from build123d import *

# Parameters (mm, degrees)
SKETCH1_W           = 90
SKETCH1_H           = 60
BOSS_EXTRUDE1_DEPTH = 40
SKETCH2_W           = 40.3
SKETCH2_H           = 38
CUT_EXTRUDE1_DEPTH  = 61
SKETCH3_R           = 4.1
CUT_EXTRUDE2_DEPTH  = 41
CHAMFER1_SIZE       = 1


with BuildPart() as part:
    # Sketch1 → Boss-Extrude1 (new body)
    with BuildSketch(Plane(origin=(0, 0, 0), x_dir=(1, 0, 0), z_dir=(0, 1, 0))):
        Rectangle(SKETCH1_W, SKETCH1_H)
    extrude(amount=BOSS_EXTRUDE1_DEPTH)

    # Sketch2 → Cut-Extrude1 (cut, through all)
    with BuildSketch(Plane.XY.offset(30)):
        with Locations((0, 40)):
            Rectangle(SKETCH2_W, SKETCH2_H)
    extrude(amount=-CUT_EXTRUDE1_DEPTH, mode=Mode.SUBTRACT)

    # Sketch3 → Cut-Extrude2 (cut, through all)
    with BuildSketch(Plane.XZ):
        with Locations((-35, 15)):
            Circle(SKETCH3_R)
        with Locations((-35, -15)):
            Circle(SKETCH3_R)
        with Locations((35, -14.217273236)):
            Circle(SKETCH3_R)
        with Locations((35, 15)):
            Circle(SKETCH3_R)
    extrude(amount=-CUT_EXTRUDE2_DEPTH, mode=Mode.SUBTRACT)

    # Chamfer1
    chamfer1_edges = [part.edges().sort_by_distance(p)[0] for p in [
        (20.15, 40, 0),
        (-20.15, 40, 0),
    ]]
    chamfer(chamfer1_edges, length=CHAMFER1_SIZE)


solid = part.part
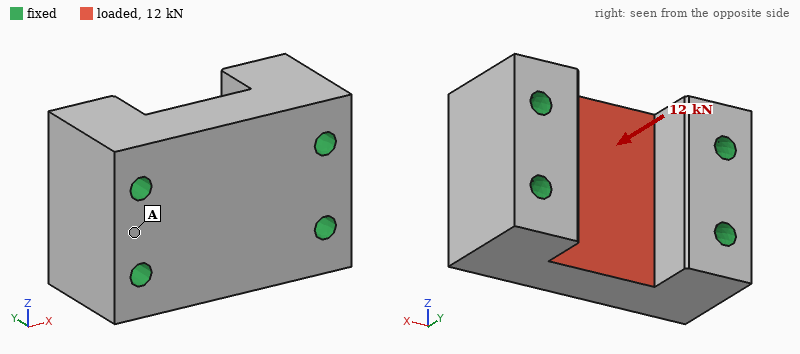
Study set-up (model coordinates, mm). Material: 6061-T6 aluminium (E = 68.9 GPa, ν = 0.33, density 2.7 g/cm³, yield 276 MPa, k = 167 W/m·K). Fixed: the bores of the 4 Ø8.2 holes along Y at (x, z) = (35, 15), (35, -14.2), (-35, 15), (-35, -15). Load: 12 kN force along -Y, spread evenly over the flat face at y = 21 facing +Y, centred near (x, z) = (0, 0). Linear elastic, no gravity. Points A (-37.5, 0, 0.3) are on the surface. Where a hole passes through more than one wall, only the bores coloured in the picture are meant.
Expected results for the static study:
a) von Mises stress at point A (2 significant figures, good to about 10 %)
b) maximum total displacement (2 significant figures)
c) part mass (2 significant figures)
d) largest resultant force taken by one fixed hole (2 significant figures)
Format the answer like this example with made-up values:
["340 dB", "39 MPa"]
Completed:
["2.6 MPa", "7.6 µm", "440 g", "3.1 kN"]
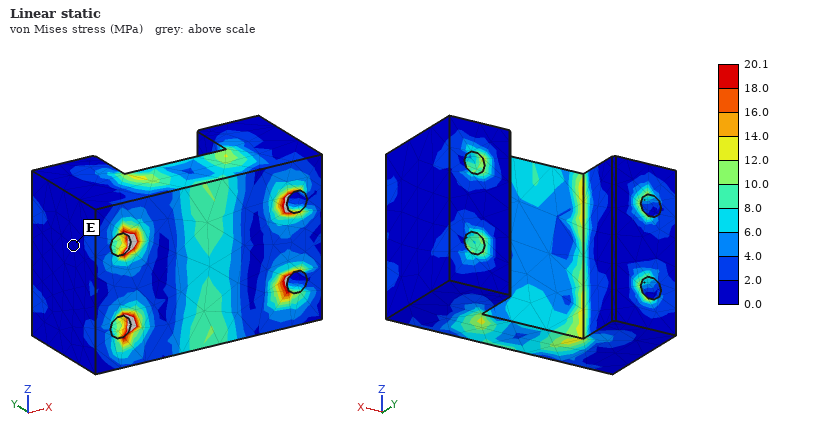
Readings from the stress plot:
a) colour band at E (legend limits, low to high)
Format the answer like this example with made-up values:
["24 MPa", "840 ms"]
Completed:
["0.0 to 2.0 MPa"]
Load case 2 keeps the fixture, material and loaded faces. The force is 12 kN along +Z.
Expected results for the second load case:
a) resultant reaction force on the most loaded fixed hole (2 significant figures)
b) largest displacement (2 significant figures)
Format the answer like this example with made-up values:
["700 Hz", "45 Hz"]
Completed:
["3.5 kN", "10 µm"]
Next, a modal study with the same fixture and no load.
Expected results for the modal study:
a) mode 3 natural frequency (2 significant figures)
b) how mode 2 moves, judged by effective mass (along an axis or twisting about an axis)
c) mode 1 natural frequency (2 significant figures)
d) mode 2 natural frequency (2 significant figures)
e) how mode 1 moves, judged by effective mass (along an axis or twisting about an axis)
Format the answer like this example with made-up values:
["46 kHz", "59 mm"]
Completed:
["22 kHz", "along Z", "19 kHz", "20 kHz", "along Y"]
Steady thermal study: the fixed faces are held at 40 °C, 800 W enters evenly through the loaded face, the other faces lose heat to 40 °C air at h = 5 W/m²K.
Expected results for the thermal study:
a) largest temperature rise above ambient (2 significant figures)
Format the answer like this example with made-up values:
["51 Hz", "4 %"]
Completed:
["53 K"]
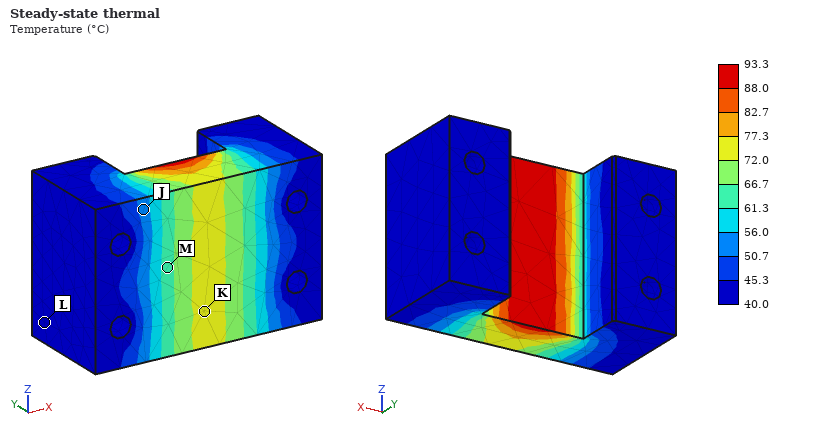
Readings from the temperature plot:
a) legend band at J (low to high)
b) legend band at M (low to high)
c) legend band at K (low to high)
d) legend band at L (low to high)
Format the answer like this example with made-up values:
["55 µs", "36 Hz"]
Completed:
["50.7 to 56.0 °C", "61.3 to 66.7 °C", "72.0 to 77.3 °C", "40.0 to 45.3 °C"]
